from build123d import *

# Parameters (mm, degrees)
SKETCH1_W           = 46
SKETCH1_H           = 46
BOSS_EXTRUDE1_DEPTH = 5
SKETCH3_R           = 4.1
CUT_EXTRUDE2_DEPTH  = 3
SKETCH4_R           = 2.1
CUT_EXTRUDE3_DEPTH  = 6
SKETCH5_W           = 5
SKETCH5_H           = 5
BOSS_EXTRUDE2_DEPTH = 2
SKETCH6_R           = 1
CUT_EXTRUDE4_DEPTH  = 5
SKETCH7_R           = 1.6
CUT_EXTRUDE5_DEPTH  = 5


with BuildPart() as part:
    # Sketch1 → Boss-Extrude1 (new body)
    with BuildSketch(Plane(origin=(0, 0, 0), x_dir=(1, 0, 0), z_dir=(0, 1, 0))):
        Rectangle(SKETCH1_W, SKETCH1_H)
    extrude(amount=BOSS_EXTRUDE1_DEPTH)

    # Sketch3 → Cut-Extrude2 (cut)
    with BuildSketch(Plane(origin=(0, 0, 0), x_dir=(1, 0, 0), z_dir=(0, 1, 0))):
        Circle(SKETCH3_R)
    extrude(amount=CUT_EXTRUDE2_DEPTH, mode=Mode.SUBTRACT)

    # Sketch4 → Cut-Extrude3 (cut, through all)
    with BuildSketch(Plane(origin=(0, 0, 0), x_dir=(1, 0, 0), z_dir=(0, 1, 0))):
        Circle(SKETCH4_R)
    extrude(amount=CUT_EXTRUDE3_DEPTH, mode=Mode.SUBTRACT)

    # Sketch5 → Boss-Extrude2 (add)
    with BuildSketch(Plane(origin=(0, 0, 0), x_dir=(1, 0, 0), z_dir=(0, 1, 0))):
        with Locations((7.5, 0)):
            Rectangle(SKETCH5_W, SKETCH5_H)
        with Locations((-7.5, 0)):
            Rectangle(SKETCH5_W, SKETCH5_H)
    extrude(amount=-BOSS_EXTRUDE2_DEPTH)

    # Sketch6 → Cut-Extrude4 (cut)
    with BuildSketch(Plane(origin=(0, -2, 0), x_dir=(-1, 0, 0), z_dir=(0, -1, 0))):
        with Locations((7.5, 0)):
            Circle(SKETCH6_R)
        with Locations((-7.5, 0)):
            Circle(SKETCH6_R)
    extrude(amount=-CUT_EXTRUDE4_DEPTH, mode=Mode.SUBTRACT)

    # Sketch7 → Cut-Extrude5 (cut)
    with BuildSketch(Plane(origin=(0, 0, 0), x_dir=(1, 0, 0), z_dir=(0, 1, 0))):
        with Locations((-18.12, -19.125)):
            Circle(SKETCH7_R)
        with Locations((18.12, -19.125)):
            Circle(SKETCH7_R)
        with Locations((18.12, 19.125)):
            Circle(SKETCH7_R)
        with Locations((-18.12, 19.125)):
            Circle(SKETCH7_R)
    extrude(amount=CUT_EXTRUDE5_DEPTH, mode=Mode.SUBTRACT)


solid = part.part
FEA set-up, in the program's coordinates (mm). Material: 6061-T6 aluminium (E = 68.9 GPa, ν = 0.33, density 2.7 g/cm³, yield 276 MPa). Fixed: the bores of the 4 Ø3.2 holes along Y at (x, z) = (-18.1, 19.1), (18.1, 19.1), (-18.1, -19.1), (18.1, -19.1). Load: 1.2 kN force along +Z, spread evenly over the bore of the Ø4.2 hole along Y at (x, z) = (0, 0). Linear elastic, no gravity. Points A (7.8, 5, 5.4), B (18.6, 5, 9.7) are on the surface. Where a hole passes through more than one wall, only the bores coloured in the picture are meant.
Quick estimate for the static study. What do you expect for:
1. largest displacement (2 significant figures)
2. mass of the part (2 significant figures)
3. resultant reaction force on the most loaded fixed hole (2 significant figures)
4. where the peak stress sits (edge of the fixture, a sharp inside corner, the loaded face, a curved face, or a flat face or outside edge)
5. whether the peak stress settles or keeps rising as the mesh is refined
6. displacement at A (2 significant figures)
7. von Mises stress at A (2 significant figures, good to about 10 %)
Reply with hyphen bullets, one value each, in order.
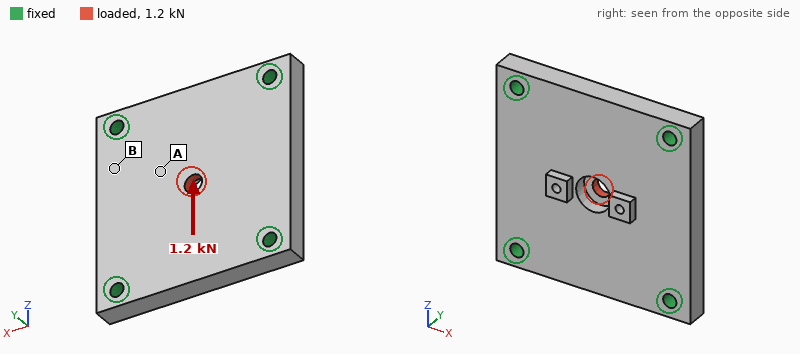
- 5.3 µm
- 28 g
- 340 N
- a sharp inside corner
- keeps rising
- 1.9 µm
- 9.2 MPa
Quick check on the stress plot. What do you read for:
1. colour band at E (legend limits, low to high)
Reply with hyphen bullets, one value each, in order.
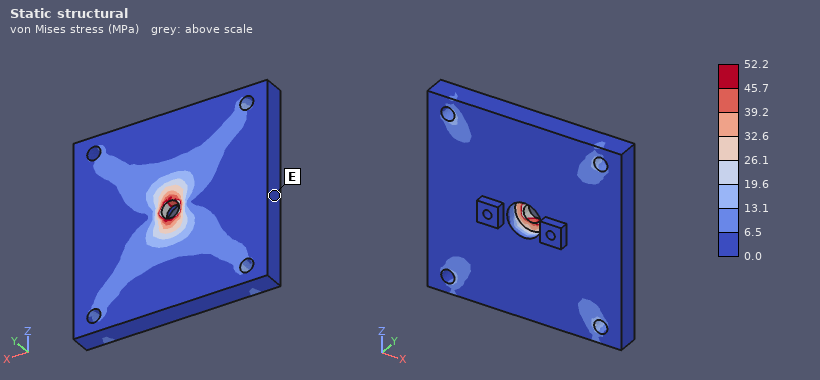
- 0.0 to 6.5 MPa
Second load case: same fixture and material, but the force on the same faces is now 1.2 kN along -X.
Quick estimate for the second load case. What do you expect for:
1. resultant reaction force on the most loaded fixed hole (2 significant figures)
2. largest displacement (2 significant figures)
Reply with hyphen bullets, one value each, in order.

- 340 N
- 5.4 µm
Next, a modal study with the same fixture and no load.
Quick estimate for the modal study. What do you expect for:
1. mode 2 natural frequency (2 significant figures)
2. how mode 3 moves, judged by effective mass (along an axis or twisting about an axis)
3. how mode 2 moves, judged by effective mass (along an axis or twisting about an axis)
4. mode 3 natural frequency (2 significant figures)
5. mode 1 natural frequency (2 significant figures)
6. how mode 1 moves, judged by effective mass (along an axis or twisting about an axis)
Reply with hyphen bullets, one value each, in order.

- 18 kHz
- twisting about X
- twisting about Z
- 19 kHz
- 11 kHz
- along Y
